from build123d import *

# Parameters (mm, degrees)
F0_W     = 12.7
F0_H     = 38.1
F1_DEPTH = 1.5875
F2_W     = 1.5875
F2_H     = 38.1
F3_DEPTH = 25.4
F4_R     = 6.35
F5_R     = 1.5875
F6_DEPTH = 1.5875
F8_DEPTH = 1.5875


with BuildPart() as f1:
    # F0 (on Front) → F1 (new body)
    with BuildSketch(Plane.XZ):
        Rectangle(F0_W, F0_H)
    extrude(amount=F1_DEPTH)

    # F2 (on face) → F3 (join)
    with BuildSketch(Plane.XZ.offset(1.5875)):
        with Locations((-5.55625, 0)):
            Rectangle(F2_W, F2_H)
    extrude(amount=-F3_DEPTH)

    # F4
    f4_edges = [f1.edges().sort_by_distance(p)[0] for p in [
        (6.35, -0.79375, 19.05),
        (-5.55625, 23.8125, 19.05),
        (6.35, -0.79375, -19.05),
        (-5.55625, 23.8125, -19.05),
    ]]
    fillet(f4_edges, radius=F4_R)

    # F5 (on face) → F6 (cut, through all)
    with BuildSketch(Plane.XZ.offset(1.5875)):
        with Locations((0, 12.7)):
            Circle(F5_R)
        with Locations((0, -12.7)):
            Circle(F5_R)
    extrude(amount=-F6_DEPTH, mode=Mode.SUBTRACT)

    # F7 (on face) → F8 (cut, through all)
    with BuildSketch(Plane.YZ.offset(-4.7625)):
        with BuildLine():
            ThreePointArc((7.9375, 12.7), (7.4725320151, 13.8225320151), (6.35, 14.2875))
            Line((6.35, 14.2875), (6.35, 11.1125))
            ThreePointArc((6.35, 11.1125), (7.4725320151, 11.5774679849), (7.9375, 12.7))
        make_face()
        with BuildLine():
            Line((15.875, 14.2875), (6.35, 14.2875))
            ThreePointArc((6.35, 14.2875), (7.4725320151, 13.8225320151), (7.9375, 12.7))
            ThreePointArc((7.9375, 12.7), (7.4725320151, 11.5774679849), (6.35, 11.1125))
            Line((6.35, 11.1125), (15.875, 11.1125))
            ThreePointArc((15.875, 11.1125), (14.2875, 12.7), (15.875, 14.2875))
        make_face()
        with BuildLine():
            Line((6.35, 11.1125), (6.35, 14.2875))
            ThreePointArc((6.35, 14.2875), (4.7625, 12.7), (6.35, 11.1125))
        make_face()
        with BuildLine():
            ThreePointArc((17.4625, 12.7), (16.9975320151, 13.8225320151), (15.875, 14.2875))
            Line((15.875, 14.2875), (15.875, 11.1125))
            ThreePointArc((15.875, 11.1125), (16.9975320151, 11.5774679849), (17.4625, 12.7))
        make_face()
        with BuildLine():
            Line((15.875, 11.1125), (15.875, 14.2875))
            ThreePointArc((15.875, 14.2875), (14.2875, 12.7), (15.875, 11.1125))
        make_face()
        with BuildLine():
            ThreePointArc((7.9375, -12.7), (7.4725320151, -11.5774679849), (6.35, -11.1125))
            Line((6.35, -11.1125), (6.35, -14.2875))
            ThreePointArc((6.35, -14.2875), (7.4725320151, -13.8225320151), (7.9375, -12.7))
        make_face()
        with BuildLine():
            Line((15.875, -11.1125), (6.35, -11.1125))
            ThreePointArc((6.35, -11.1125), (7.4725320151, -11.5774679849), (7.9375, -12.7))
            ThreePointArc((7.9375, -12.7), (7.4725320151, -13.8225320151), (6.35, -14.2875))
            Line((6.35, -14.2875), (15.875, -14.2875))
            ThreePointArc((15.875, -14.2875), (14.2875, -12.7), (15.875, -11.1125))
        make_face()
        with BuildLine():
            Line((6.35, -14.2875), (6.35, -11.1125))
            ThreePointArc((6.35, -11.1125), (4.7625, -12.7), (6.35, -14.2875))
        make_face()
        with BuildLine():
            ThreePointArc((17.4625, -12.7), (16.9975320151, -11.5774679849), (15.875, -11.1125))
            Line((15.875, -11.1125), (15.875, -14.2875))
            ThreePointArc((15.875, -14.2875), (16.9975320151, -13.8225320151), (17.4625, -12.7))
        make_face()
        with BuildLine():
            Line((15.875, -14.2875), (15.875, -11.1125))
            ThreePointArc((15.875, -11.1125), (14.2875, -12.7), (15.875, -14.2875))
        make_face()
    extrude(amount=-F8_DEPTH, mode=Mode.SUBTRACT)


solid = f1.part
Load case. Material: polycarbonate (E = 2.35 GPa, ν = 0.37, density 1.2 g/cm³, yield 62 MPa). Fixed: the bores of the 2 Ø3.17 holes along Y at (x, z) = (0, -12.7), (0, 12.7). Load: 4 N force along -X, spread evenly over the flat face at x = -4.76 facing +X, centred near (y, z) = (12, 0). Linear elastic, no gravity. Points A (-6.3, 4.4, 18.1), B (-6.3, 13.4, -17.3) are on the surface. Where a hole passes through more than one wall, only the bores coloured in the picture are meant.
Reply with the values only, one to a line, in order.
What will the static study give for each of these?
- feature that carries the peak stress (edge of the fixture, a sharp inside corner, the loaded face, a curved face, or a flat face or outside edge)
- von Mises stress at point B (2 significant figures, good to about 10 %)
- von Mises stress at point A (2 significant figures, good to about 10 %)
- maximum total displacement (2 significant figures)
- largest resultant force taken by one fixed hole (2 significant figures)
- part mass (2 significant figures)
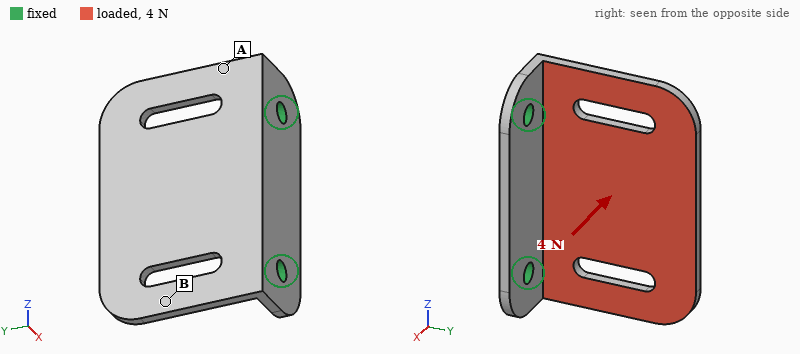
a flat face or outside edge
0.77 MPa
2.2 MPa
0.46 mm
2.0 N
2.4 g
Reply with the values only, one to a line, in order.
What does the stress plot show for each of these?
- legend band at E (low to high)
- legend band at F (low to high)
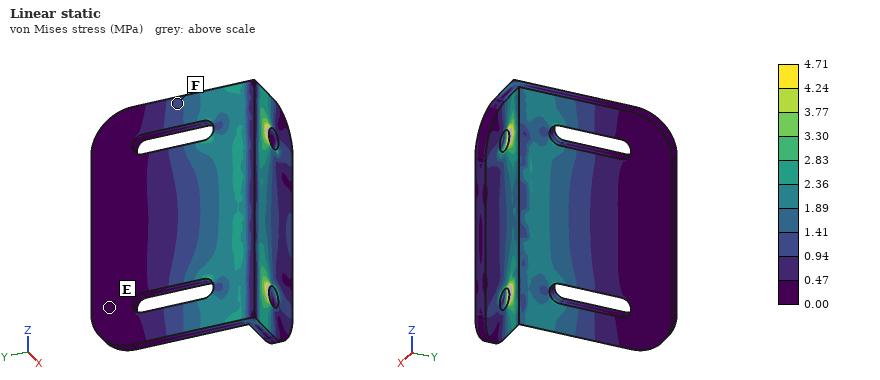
0.00 to 0.47 MPa
0.94 to 1.41 MPa
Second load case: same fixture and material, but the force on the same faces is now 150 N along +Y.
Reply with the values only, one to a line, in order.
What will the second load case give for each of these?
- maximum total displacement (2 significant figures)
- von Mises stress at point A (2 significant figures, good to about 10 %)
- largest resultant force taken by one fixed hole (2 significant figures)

0.56 mm
5.3 MPa
76 N
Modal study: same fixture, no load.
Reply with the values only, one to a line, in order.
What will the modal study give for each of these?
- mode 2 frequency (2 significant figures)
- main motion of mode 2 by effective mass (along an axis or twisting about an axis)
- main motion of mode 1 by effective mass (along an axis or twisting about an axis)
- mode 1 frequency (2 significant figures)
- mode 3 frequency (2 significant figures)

980 Hz
twisting about Y
along X
470 Hz
2200 Hz
